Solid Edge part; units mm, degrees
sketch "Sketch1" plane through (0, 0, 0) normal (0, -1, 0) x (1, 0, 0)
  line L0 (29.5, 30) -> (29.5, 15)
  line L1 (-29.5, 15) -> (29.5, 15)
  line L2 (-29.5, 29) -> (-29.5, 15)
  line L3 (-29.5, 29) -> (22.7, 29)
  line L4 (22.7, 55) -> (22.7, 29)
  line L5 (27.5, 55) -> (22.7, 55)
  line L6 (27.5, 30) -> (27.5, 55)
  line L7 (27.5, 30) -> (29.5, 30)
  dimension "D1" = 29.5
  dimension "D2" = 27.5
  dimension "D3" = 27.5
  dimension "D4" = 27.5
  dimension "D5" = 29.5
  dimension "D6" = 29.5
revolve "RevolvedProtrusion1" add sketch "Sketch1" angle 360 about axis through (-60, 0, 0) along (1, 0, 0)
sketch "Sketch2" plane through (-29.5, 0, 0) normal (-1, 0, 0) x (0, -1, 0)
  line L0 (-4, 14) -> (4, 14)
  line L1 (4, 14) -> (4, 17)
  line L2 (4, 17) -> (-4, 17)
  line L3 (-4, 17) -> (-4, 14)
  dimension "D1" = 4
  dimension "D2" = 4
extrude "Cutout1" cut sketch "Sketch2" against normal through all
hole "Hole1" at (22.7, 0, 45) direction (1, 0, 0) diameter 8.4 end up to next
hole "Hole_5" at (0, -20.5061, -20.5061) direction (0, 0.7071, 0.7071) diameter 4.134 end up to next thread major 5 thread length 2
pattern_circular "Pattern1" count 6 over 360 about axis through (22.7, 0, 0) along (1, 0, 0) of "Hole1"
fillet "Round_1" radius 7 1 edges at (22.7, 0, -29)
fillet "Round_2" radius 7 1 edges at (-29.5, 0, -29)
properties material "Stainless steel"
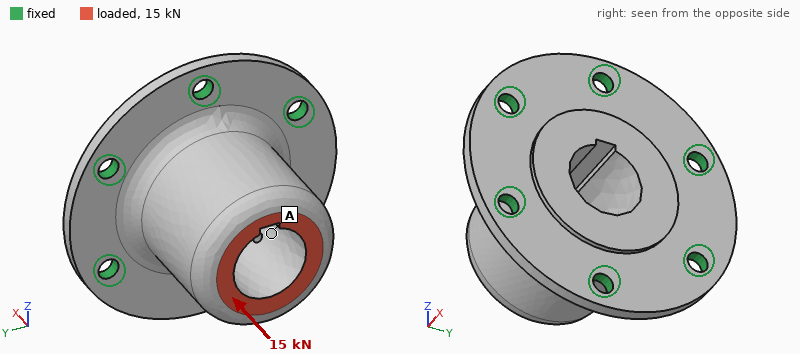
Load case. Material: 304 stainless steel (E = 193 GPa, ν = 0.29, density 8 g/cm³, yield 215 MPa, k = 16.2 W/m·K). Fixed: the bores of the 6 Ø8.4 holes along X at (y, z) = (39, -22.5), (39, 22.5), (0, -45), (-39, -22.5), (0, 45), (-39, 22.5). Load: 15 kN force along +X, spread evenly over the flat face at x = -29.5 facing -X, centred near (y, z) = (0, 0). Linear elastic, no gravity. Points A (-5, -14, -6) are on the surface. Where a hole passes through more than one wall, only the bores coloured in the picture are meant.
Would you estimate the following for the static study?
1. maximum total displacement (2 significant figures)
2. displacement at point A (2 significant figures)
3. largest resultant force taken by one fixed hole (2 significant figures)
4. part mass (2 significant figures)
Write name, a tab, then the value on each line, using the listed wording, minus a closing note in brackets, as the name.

maximum total displacement	18 µm
displacement at point A	16 µm
largest resultant force taken by one fixed hole	2.9 kN
part mass	1.2 kg
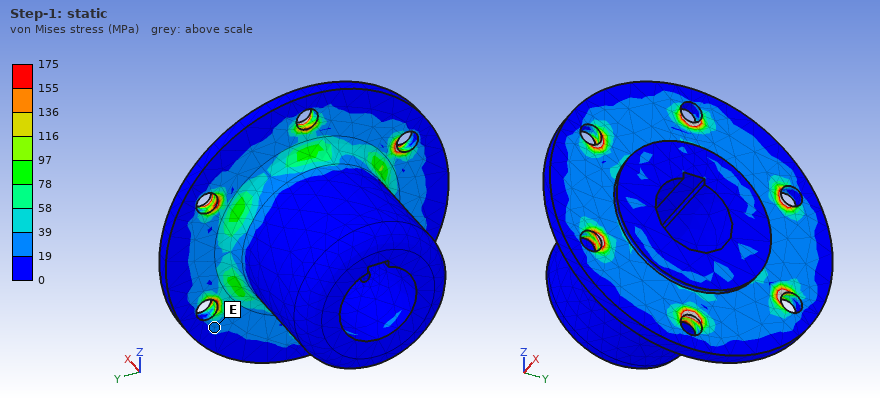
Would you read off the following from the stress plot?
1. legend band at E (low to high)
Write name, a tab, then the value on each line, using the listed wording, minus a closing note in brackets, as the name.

legend band at E	19 to 39 MPa
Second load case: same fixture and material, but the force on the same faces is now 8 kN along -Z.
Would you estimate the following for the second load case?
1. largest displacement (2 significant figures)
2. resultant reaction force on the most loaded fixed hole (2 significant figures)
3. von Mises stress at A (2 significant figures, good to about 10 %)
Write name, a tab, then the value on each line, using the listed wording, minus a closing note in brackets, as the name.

largest displacement	43 µm
resultant reaction force on the most loaded fixed hole	4.4 kN
von Mises stress at A	17 MPa
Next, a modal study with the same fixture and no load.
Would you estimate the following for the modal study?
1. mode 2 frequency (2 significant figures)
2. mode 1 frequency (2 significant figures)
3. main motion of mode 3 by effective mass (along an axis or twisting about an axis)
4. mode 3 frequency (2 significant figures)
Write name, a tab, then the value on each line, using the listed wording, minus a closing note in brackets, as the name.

mode 2 frequency	4000 Hz
mode 1 frequency	4000 Hz
main motion of mode 3 by effective mass	along X
mode 3 frequency	5100 Hz
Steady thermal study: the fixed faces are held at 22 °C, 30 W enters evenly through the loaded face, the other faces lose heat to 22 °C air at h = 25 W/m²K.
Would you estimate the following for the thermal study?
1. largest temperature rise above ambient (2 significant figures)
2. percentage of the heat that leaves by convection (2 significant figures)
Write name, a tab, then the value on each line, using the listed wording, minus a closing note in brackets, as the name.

largest temperature rise above ambient	61 K
percentage of the heat that leaves by convection	54 %
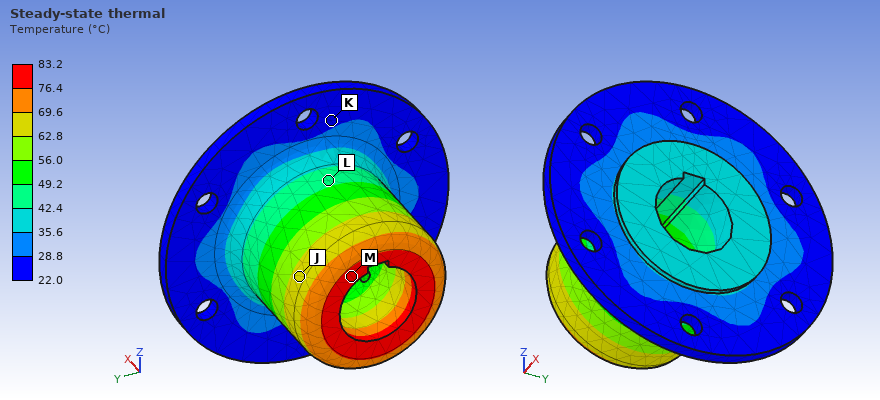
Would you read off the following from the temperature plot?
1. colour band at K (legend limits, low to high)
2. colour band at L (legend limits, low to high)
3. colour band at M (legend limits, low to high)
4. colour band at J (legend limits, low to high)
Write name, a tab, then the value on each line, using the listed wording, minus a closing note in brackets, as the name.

colour band at K	22.0 to 28.8 °C
colour band at L	42.4 to 49.2 °C
colour band at M	76.4 to 83.2 °C
colour band at J	62.8 to 69.6 °C
